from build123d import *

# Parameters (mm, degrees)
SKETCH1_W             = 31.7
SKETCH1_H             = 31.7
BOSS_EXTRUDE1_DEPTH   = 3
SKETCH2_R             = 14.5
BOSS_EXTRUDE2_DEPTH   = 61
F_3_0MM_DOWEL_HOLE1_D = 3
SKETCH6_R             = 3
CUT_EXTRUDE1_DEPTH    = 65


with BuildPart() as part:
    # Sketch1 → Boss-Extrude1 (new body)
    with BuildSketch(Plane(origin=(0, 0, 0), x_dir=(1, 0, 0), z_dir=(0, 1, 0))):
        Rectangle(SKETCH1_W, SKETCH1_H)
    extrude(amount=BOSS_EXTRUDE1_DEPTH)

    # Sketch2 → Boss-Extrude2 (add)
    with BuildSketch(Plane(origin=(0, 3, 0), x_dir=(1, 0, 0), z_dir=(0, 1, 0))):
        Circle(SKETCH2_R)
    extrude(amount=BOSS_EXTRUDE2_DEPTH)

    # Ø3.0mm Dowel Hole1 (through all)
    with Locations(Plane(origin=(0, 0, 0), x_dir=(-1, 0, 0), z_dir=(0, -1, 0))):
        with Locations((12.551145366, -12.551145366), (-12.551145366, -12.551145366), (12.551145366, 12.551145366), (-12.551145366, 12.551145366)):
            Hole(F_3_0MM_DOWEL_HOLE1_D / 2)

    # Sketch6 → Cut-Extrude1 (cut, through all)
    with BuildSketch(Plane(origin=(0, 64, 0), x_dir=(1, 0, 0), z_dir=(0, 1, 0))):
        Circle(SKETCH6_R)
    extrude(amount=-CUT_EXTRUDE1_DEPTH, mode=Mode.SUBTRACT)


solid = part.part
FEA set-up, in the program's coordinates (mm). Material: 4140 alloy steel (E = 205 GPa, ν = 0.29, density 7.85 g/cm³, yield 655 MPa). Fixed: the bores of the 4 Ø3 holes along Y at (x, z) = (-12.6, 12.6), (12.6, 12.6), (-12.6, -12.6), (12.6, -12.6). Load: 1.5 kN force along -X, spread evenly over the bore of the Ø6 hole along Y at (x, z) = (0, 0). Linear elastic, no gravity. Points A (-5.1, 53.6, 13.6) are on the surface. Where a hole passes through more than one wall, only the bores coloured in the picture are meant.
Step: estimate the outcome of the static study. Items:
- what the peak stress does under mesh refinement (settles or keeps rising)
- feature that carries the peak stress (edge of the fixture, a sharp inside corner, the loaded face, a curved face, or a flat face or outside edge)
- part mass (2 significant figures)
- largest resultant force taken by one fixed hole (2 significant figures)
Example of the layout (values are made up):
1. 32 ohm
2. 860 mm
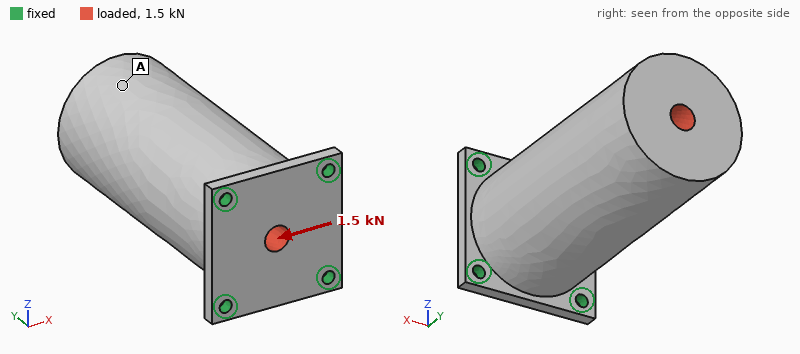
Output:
1. keeps rising
2. edge of the fixture
3. 330 g
4. 1.1 kN
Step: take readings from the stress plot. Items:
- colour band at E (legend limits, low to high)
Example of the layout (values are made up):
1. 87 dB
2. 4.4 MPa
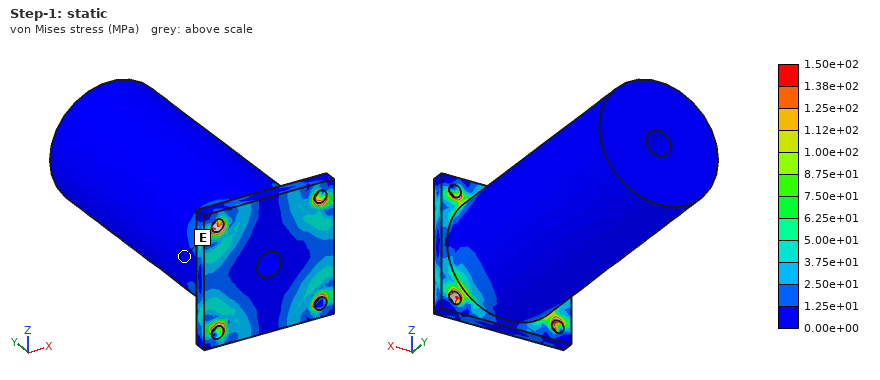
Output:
1. 0.00e+00 to 1.25e+01 MPa
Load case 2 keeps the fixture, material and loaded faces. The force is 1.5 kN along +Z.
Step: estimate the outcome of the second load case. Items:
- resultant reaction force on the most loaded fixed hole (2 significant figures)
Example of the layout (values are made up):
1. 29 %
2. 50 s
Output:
1. 1.1 kN
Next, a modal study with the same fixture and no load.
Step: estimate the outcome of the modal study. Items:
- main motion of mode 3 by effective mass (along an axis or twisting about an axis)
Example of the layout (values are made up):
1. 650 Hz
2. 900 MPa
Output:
1. along Y
